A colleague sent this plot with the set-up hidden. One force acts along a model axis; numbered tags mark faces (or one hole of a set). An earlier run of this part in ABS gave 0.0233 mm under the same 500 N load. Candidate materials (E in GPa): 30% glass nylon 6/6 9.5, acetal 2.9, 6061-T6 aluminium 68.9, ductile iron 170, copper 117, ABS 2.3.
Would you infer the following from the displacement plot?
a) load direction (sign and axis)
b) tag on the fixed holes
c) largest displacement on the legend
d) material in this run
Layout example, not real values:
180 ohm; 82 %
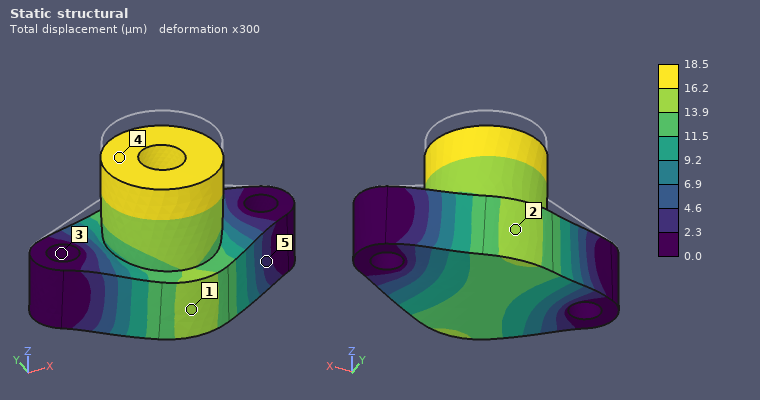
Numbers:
-Z; 3; 18.5 µm; acetal
